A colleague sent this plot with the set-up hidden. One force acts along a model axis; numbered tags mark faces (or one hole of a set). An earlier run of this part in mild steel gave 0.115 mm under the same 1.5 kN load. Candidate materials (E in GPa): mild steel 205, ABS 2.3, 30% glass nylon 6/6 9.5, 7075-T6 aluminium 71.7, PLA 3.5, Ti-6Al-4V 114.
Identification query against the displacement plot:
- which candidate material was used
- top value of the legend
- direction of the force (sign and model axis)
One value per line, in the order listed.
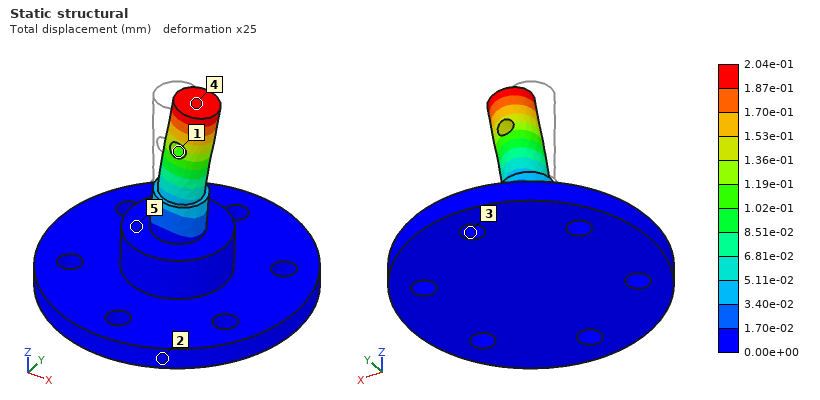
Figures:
Ti-6Al-4V
2.04e-01 mm
+X
